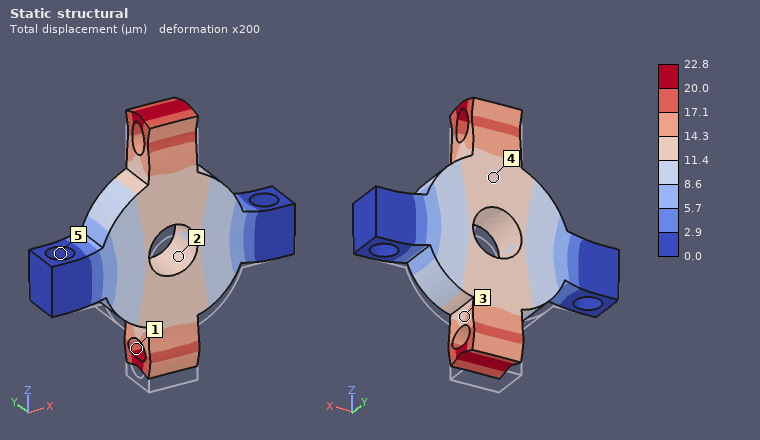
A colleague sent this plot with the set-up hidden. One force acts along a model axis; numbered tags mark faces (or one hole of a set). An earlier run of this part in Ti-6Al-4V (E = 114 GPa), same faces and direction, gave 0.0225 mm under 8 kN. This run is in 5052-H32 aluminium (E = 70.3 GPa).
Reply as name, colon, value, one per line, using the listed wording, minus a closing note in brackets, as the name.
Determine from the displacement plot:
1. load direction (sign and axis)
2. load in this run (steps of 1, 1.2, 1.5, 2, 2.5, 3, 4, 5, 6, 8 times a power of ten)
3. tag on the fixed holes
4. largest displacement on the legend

load direction: +Z
load in this run: 5 kN
tag on the fixed holes: 5
largest displacement on the legend: 22.8 µm
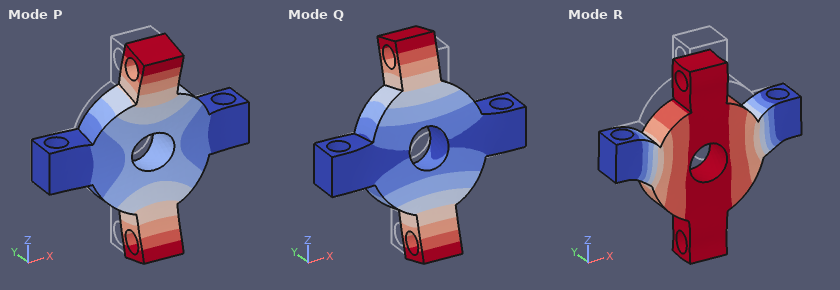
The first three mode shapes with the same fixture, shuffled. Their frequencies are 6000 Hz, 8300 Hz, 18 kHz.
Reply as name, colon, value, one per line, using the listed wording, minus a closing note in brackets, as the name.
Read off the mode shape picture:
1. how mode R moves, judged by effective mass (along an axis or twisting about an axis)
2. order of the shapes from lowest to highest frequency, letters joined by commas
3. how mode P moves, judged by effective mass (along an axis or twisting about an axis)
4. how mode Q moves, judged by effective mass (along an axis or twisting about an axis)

how mode R moves, judged by effective mass: along Z
order of the shapes from lowest to highest frequency, letters joined by commas: Q, P, R
how mode P moves, judged by effective mass: along Y
how mode Q moves, judged by effective mass: twisting about X
